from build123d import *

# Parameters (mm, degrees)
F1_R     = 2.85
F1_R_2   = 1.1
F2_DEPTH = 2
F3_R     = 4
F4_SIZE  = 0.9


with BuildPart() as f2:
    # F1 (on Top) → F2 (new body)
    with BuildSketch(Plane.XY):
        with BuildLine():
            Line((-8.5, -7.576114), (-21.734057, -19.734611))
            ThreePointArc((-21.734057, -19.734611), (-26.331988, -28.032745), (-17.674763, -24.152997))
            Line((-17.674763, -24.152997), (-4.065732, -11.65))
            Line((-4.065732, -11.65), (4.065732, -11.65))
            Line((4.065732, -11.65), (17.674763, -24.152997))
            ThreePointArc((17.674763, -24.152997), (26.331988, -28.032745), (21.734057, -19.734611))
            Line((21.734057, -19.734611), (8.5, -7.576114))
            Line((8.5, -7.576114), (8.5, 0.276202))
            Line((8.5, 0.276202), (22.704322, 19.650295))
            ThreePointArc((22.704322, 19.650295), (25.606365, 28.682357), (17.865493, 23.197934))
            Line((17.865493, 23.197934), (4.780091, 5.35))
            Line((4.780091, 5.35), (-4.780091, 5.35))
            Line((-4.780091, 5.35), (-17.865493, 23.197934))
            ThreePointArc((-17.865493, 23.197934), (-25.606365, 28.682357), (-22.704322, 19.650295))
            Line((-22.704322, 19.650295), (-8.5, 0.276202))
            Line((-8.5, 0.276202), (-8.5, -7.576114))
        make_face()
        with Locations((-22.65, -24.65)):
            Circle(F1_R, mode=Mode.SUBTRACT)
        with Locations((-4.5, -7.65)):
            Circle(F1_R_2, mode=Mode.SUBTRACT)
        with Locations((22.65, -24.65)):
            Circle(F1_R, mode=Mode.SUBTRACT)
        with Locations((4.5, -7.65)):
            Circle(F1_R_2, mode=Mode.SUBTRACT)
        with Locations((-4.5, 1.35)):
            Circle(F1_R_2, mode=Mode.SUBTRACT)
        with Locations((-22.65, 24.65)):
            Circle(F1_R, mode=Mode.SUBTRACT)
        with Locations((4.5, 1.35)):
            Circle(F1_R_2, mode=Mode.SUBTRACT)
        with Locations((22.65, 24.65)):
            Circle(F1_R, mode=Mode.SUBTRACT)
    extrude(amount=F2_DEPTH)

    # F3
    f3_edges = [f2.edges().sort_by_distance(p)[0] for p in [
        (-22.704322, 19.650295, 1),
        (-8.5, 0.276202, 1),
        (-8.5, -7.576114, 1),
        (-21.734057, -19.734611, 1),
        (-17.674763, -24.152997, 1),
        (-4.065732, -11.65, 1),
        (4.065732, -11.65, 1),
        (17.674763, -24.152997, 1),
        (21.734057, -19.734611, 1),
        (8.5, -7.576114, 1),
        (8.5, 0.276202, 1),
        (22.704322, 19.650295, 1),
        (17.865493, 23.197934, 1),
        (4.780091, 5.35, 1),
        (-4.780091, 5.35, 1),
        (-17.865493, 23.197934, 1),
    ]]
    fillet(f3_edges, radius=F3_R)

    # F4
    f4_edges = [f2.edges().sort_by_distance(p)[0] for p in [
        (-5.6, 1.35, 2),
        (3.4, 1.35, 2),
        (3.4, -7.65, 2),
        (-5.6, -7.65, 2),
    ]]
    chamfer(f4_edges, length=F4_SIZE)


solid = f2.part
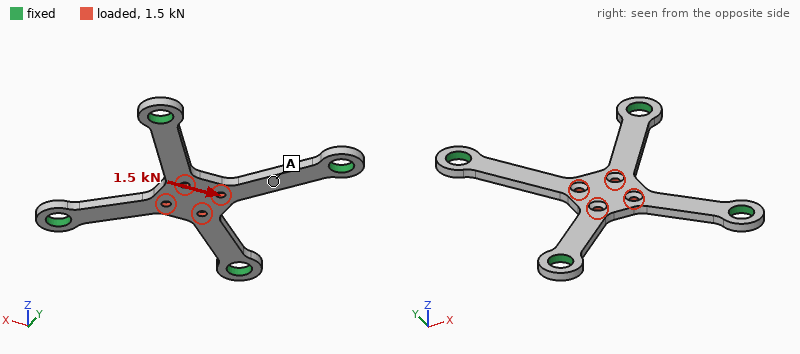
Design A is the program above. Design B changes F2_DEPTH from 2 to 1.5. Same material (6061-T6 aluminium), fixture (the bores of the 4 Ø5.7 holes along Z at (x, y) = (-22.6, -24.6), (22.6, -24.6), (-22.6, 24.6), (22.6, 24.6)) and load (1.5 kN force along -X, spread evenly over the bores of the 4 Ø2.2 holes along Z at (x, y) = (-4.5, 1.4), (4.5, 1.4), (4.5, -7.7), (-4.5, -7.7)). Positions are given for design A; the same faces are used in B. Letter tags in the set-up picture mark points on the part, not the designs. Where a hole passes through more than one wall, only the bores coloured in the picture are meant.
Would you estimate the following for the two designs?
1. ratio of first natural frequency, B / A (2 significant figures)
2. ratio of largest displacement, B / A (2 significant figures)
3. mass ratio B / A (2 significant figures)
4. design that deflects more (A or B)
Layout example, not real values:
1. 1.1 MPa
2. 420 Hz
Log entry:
1. 0.76
2. 1.9
3. 0.75
4. B
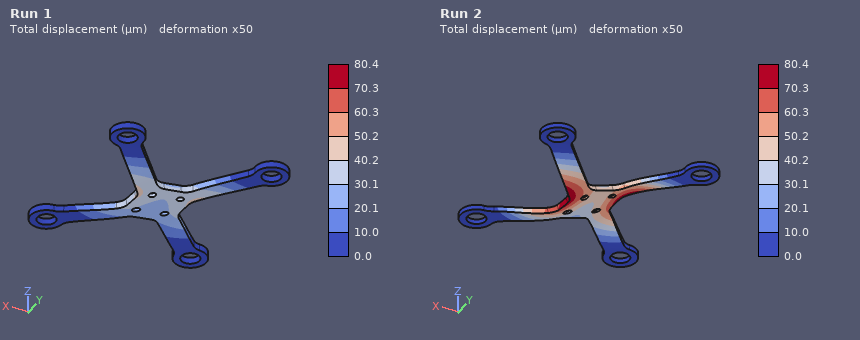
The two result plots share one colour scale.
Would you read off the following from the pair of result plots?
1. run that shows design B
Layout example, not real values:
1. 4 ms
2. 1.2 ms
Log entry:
1. Run 2
